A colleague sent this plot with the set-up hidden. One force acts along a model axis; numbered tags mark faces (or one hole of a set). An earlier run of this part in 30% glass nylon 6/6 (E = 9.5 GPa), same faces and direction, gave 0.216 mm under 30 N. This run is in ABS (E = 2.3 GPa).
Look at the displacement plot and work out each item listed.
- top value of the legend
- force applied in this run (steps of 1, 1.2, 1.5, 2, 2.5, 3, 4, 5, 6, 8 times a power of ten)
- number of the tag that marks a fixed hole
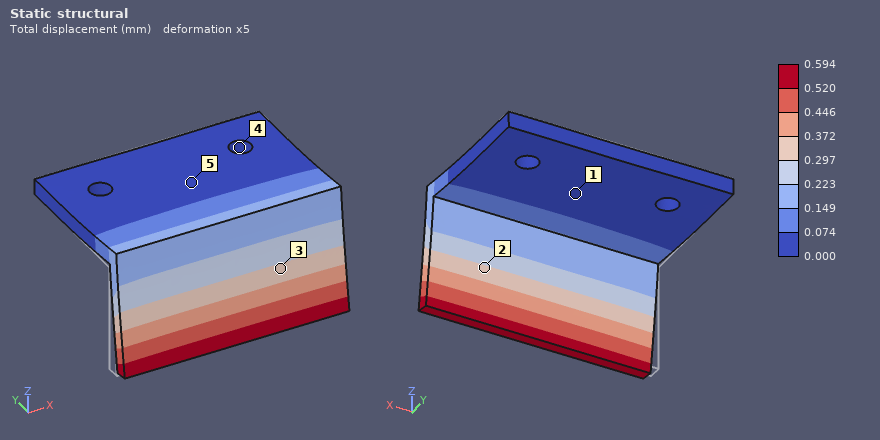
0.594 mm
20 N
4
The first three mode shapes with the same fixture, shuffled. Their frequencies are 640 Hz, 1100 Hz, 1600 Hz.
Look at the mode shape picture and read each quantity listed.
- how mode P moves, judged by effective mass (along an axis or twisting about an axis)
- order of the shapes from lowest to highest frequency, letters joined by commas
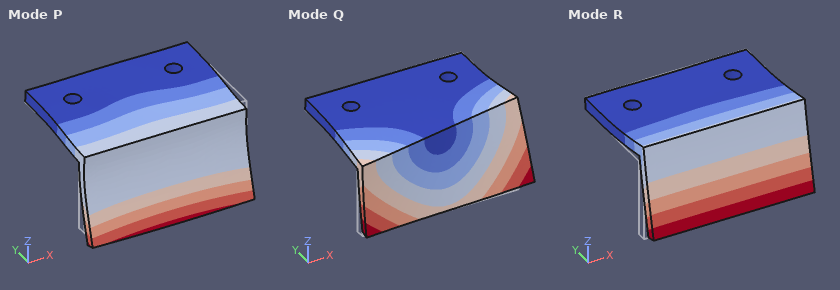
along Z
R, Q, P
